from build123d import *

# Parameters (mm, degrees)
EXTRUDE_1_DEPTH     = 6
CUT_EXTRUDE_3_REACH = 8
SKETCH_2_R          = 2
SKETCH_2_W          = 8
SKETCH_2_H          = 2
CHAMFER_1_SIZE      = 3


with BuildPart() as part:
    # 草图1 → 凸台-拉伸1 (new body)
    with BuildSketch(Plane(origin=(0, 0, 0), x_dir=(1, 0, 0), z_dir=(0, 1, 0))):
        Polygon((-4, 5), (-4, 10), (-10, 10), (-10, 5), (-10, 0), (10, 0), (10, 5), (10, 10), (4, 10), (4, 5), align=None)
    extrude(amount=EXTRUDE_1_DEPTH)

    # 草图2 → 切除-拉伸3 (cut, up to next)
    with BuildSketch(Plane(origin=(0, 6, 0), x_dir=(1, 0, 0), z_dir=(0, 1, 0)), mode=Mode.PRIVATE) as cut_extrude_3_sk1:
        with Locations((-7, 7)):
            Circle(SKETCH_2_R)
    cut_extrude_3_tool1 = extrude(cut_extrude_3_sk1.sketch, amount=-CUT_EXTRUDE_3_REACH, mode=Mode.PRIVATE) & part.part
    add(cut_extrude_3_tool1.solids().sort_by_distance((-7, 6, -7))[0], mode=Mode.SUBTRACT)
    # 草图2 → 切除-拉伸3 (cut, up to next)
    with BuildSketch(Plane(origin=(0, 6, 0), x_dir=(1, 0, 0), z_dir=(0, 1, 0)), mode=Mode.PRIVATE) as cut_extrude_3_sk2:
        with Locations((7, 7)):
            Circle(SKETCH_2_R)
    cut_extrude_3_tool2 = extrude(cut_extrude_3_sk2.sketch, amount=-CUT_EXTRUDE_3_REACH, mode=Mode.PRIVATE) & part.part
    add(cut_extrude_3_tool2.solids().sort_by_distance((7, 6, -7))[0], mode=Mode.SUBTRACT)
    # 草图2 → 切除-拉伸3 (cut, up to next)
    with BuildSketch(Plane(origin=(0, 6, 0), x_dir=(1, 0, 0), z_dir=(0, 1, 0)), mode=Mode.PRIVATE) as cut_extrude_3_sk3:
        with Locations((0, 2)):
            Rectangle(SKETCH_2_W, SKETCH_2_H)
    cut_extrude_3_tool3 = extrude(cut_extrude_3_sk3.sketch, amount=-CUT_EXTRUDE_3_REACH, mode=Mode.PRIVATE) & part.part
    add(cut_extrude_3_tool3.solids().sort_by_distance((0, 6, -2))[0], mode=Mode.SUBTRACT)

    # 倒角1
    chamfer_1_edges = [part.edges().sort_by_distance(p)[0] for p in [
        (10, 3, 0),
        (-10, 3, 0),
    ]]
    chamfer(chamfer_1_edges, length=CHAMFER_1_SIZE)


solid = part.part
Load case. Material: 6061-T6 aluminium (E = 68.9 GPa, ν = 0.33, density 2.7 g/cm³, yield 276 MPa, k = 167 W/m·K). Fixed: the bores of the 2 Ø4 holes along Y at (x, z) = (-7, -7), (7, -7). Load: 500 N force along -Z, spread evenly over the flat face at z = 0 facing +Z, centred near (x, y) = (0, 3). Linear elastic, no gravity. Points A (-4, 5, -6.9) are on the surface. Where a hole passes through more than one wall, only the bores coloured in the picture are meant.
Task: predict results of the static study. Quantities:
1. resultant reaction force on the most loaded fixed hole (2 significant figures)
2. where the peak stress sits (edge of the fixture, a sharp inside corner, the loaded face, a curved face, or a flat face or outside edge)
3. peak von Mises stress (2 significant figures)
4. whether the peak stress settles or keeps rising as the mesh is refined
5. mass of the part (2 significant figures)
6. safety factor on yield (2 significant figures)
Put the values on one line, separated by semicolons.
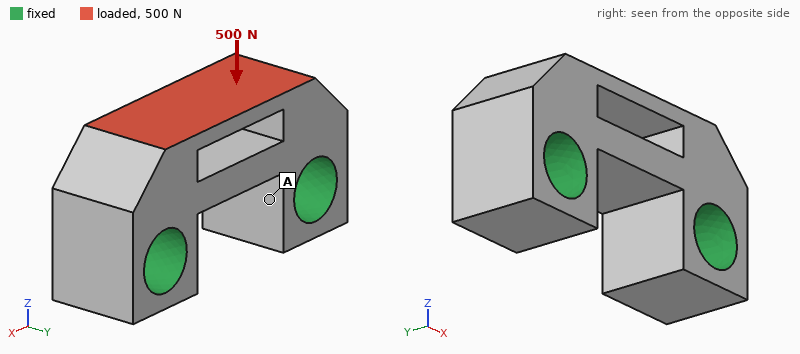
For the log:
270 N; the loaded face; 130 MPa; settles; 1.8 g; 2.1
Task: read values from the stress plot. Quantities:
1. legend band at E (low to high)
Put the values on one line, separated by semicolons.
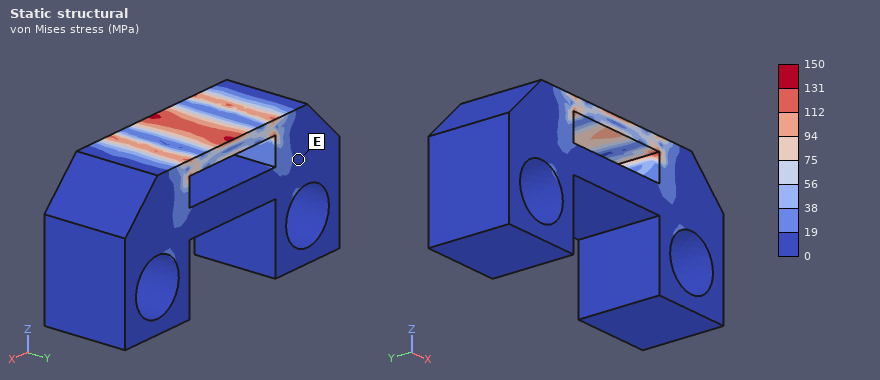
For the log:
0 to 19 MPa
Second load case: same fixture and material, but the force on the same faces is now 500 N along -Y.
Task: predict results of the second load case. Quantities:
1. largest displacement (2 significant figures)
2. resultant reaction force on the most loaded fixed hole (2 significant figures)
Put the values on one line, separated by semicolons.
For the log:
13 µm; 250 N
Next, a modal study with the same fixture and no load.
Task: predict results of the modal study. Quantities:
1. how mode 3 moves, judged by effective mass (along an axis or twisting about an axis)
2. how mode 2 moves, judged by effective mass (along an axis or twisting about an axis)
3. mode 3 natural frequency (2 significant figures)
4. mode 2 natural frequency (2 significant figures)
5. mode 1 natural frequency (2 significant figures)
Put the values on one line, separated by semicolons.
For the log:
along Y; along Y; 81 kHz; 75 kHz; 59 kHz
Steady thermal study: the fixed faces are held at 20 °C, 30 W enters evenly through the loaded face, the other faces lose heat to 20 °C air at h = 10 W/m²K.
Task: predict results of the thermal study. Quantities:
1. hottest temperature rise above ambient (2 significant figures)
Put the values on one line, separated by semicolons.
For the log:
40 K
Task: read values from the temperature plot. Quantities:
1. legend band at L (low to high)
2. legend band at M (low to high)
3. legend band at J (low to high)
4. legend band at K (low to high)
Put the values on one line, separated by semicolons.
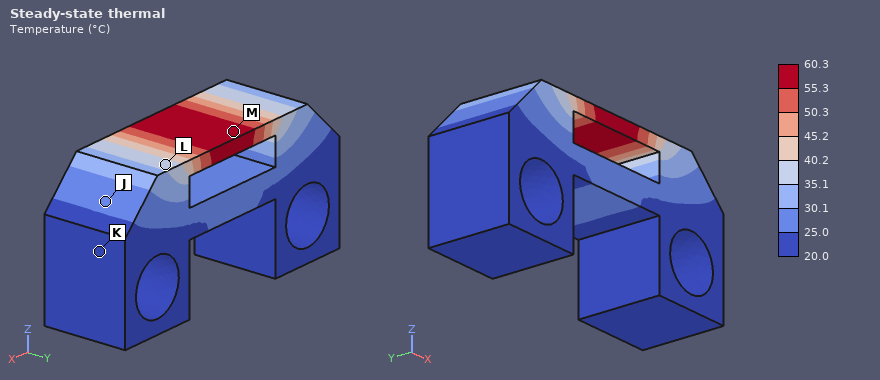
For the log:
35.1 to 40.2 °C; 55.3 to 60.3 °C; 25.0 to 30.1 °C; 20.0 to 25.0 °C
